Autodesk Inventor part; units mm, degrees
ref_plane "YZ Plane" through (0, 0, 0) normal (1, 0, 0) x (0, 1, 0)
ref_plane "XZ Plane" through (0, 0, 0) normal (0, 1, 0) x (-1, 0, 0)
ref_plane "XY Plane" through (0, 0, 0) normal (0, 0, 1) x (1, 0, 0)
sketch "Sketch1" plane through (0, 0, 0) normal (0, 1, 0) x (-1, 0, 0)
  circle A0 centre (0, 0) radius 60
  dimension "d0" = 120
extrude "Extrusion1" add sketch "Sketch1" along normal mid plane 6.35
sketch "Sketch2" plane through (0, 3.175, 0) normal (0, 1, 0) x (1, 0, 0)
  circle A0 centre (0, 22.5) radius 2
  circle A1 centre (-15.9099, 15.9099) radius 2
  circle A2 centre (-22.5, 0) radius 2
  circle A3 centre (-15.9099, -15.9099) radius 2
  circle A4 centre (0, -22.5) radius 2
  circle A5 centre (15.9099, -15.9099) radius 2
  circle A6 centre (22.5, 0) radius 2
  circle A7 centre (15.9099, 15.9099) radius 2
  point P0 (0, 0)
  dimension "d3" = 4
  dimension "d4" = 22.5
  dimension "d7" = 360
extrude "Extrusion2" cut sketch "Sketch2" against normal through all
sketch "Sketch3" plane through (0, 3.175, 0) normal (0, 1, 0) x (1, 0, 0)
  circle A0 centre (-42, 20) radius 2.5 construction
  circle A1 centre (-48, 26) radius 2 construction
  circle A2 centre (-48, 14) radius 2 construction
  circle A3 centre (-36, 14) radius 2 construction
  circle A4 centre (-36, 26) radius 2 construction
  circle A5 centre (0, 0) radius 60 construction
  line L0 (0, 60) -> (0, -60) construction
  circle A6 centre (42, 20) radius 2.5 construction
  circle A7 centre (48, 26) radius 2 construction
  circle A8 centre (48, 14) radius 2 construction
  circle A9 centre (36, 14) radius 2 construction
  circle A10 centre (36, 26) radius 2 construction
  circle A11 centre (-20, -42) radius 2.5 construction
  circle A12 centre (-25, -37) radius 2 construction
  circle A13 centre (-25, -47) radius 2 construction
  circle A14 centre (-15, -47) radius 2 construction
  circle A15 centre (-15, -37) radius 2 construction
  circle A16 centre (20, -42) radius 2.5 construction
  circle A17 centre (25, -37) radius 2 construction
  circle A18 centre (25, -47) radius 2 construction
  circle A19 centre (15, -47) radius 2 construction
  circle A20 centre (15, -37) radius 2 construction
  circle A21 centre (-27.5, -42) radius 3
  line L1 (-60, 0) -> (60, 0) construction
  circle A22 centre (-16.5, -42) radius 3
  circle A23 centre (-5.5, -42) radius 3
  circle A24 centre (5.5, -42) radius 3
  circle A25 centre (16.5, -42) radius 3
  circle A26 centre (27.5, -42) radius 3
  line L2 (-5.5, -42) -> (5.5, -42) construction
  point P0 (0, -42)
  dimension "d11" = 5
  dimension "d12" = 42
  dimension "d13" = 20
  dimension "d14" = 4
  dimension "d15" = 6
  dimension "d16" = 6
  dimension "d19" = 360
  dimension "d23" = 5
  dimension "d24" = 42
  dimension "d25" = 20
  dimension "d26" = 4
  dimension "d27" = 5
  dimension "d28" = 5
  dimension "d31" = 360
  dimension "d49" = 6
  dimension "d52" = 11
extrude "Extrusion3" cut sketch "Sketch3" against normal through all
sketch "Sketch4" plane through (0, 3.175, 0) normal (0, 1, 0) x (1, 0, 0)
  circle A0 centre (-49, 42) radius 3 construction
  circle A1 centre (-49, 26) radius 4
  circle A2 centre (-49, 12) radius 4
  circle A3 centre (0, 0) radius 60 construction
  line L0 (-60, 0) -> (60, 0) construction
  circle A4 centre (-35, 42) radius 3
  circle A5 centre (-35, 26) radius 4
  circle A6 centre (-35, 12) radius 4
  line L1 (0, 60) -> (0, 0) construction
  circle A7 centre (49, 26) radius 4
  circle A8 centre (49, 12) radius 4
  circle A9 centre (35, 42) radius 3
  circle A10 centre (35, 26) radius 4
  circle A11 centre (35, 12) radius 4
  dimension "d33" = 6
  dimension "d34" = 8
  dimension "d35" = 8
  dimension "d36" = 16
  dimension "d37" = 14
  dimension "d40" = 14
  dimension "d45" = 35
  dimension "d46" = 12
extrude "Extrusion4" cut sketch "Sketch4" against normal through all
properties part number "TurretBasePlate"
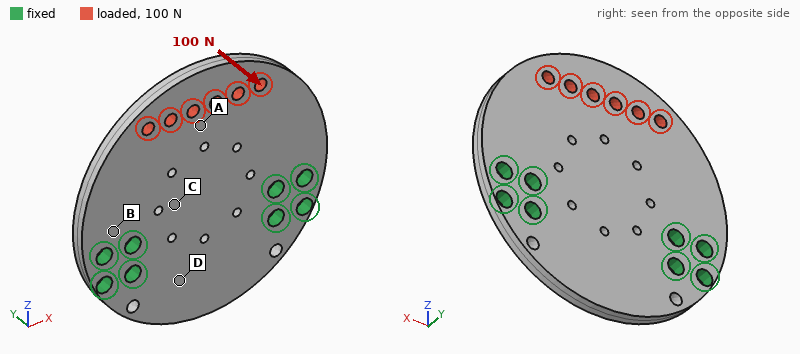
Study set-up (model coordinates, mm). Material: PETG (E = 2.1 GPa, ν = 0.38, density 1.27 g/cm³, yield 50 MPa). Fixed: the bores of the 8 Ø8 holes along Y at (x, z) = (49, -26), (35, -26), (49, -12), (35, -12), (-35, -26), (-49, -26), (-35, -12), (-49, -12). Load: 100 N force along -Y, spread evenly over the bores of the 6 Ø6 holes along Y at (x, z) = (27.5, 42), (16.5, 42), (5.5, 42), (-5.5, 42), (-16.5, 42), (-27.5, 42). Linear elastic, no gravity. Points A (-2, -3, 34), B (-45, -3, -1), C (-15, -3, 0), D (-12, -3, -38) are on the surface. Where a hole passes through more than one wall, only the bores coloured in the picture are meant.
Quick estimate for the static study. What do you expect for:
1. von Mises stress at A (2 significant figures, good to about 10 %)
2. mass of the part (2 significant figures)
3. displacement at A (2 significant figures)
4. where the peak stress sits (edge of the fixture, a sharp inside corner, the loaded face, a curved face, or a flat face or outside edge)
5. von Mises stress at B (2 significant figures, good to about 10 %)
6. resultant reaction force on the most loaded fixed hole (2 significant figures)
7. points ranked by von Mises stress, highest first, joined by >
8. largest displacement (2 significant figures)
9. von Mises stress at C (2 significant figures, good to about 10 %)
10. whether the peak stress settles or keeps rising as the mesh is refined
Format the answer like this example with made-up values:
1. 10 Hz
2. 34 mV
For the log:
1. 2.1 MPa
2. 85 g
3. 0.91 mm
4. edge of the fixture
5. 5.9 MPa
6. 100 N
7. B > C > A > D
8. 1.7 mm
9. 4.4 MPa
10. keeps rising
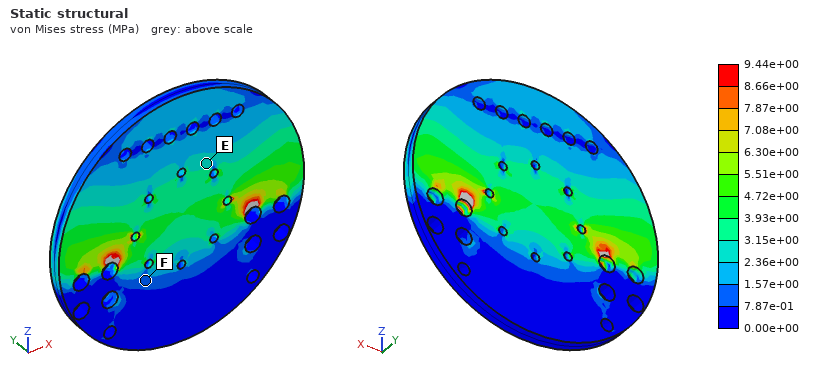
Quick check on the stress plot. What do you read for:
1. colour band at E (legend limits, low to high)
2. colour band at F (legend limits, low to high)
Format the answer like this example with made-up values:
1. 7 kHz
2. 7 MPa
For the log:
1. 2.36e+00 to 3.15e+00 MPa
2. 7.87e-01 to 1.57e+00 MPa
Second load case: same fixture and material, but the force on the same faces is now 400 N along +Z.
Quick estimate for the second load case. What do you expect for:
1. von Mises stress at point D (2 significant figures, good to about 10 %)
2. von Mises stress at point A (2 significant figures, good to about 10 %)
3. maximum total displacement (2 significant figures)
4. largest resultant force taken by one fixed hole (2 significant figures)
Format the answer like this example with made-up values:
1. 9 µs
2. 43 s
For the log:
1. 0.21 MPa
2. 0.73 MPa
3. 28 µm
4. 97 N
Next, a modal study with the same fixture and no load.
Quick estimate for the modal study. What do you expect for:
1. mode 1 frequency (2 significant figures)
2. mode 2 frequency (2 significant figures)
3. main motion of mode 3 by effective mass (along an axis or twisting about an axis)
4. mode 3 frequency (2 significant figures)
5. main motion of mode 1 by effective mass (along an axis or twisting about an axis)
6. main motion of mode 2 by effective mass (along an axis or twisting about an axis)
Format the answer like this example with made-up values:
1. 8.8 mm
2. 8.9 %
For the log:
1. 330 Hz
2. 740 Hz
3. along Y
4. 1100 Hz
5. along Y
6. twisting about Z
